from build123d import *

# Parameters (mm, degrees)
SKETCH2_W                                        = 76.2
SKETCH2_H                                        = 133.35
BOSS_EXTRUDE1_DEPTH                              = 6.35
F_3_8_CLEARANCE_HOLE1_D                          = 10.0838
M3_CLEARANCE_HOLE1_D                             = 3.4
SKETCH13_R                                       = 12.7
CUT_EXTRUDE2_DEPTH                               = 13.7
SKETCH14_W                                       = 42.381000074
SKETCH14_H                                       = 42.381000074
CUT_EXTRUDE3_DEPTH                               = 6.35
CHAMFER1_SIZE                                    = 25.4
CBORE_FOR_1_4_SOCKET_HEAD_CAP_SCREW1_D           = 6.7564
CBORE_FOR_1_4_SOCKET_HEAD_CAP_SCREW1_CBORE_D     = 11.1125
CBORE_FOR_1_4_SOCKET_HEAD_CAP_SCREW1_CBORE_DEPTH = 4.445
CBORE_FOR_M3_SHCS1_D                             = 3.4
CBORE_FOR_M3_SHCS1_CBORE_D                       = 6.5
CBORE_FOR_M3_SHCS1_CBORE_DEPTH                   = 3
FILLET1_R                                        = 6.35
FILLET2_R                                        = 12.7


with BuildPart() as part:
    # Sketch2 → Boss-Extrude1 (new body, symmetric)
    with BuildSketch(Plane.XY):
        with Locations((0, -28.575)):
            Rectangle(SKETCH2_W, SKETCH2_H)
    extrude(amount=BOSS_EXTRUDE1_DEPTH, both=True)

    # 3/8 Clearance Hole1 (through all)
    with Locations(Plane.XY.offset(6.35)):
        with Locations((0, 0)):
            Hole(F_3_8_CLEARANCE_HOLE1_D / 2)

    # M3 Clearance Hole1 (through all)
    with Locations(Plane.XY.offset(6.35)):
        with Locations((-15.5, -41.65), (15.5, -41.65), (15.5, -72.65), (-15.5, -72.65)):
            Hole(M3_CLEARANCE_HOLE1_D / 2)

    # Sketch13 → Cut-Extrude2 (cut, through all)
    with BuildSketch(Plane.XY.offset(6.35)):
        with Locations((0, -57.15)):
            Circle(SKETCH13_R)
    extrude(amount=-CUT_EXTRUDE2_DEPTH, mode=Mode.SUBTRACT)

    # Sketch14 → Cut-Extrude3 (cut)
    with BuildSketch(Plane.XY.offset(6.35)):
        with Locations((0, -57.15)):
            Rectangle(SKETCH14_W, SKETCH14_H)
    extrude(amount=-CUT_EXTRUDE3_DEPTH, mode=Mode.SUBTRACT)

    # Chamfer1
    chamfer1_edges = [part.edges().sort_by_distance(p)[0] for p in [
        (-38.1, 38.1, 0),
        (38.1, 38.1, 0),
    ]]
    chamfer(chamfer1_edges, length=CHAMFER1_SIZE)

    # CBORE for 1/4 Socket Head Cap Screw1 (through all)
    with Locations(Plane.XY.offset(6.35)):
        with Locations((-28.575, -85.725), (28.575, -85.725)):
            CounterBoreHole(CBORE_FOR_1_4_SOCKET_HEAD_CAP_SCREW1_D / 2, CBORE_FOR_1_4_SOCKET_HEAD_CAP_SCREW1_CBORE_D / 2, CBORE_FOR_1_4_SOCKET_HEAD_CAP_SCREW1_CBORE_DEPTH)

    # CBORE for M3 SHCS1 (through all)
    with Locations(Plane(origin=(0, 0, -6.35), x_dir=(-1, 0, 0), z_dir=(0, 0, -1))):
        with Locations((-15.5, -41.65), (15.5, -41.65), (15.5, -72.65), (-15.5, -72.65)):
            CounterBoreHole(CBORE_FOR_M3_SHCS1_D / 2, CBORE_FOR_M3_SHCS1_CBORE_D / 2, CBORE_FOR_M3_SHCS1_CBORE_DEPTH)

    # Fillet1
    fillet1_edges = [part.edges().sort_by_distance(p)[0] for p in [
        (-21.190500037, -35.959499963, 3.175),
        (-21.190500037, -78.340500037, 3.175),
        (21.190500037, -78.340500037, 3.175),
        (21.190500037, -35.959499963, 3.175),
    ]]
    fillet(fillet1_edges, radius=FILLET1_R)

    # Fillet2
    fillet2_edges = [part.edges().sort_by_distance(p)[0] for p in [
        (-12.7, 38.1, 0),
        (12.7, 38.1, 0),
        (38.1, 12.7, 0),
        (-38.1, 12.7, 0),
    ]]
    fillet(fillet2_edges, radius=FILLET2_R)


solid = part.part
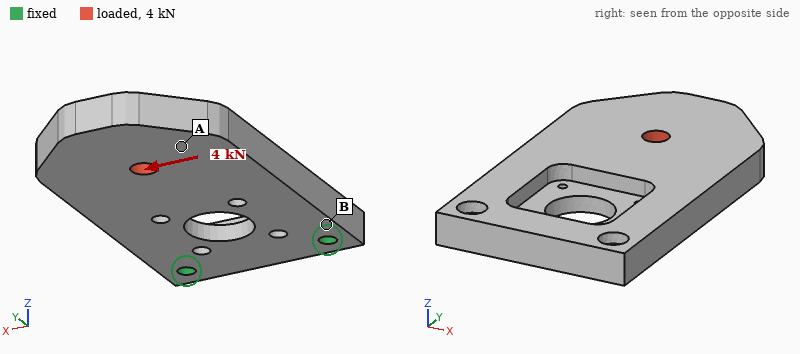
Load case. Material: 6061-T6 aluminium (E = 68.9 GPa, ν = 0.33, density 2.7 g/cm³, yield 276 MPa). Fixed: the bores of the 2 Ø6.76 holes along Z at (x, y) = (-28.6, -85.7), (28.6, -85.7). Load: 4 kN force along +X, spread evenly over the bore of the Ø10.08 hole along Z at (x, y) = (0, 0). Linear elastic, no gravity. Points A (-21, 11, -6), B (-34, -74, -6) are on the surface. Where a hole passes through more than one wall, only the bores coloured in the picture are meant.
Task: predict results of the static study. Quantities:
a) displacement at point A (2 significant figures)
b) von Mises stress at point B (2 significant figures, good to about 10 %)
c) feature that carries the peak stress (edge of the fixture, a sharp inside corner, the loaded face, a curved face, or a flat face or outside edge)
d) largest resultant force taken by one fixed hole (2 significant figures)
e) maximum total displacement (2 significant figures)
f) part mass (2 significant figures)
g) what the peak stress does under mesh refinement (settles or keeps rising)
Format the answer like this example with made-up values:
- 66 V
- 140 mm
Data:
- 77 µm
- 40 MPa
- edge of the fixture
- 5.9 kN
- 96 µm
- 280 g
- keeps rising
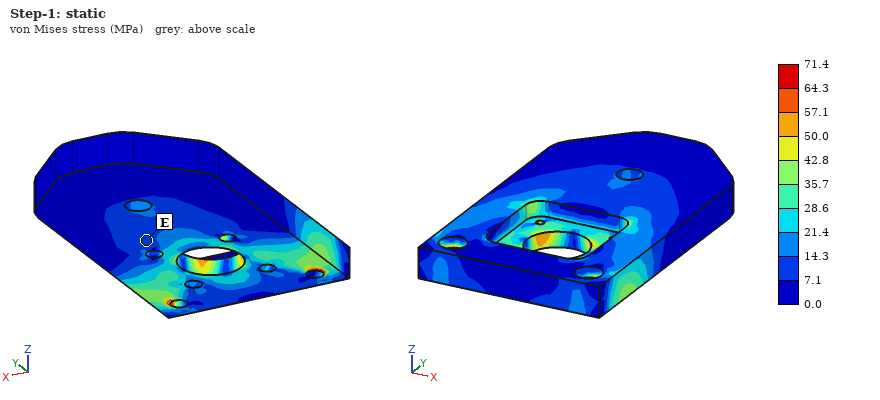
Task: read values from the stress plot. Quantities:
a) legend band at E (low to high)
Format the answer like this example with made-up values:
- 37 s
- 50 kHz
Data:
- 7.1 to 14.3 MPa
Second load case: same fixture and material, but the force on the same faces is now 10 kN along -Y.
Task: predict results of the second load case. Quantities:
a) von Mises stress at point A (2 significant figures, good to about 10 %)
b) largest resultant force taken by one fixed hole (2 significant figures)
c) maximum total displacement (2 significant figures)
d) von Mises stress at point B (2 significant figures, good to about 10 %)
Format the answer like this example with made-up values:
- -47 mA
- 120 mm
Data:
- 7.3 MPa
- 5.0 kN
- 0.14 mm
- 14 MPa
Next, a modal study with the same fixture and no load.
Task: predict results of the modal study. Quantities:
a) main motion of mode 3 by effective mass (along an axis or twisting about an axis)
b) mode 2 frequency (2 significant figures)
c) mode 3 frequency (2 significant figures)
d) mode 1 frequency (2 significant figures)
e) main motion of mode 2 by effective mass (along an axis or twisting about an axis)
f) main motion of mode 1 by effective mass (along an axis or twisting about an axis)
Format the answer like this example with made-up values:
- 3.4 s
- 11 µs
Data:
- along X
- 2100 Hz
- 2800 Hz
- 520 Hz
- twisting about Y
- along Z
